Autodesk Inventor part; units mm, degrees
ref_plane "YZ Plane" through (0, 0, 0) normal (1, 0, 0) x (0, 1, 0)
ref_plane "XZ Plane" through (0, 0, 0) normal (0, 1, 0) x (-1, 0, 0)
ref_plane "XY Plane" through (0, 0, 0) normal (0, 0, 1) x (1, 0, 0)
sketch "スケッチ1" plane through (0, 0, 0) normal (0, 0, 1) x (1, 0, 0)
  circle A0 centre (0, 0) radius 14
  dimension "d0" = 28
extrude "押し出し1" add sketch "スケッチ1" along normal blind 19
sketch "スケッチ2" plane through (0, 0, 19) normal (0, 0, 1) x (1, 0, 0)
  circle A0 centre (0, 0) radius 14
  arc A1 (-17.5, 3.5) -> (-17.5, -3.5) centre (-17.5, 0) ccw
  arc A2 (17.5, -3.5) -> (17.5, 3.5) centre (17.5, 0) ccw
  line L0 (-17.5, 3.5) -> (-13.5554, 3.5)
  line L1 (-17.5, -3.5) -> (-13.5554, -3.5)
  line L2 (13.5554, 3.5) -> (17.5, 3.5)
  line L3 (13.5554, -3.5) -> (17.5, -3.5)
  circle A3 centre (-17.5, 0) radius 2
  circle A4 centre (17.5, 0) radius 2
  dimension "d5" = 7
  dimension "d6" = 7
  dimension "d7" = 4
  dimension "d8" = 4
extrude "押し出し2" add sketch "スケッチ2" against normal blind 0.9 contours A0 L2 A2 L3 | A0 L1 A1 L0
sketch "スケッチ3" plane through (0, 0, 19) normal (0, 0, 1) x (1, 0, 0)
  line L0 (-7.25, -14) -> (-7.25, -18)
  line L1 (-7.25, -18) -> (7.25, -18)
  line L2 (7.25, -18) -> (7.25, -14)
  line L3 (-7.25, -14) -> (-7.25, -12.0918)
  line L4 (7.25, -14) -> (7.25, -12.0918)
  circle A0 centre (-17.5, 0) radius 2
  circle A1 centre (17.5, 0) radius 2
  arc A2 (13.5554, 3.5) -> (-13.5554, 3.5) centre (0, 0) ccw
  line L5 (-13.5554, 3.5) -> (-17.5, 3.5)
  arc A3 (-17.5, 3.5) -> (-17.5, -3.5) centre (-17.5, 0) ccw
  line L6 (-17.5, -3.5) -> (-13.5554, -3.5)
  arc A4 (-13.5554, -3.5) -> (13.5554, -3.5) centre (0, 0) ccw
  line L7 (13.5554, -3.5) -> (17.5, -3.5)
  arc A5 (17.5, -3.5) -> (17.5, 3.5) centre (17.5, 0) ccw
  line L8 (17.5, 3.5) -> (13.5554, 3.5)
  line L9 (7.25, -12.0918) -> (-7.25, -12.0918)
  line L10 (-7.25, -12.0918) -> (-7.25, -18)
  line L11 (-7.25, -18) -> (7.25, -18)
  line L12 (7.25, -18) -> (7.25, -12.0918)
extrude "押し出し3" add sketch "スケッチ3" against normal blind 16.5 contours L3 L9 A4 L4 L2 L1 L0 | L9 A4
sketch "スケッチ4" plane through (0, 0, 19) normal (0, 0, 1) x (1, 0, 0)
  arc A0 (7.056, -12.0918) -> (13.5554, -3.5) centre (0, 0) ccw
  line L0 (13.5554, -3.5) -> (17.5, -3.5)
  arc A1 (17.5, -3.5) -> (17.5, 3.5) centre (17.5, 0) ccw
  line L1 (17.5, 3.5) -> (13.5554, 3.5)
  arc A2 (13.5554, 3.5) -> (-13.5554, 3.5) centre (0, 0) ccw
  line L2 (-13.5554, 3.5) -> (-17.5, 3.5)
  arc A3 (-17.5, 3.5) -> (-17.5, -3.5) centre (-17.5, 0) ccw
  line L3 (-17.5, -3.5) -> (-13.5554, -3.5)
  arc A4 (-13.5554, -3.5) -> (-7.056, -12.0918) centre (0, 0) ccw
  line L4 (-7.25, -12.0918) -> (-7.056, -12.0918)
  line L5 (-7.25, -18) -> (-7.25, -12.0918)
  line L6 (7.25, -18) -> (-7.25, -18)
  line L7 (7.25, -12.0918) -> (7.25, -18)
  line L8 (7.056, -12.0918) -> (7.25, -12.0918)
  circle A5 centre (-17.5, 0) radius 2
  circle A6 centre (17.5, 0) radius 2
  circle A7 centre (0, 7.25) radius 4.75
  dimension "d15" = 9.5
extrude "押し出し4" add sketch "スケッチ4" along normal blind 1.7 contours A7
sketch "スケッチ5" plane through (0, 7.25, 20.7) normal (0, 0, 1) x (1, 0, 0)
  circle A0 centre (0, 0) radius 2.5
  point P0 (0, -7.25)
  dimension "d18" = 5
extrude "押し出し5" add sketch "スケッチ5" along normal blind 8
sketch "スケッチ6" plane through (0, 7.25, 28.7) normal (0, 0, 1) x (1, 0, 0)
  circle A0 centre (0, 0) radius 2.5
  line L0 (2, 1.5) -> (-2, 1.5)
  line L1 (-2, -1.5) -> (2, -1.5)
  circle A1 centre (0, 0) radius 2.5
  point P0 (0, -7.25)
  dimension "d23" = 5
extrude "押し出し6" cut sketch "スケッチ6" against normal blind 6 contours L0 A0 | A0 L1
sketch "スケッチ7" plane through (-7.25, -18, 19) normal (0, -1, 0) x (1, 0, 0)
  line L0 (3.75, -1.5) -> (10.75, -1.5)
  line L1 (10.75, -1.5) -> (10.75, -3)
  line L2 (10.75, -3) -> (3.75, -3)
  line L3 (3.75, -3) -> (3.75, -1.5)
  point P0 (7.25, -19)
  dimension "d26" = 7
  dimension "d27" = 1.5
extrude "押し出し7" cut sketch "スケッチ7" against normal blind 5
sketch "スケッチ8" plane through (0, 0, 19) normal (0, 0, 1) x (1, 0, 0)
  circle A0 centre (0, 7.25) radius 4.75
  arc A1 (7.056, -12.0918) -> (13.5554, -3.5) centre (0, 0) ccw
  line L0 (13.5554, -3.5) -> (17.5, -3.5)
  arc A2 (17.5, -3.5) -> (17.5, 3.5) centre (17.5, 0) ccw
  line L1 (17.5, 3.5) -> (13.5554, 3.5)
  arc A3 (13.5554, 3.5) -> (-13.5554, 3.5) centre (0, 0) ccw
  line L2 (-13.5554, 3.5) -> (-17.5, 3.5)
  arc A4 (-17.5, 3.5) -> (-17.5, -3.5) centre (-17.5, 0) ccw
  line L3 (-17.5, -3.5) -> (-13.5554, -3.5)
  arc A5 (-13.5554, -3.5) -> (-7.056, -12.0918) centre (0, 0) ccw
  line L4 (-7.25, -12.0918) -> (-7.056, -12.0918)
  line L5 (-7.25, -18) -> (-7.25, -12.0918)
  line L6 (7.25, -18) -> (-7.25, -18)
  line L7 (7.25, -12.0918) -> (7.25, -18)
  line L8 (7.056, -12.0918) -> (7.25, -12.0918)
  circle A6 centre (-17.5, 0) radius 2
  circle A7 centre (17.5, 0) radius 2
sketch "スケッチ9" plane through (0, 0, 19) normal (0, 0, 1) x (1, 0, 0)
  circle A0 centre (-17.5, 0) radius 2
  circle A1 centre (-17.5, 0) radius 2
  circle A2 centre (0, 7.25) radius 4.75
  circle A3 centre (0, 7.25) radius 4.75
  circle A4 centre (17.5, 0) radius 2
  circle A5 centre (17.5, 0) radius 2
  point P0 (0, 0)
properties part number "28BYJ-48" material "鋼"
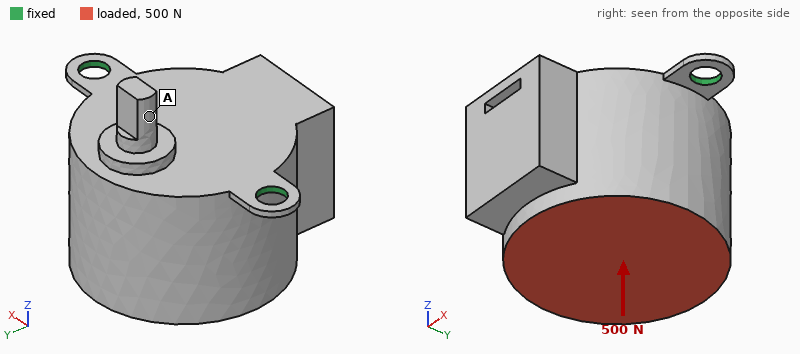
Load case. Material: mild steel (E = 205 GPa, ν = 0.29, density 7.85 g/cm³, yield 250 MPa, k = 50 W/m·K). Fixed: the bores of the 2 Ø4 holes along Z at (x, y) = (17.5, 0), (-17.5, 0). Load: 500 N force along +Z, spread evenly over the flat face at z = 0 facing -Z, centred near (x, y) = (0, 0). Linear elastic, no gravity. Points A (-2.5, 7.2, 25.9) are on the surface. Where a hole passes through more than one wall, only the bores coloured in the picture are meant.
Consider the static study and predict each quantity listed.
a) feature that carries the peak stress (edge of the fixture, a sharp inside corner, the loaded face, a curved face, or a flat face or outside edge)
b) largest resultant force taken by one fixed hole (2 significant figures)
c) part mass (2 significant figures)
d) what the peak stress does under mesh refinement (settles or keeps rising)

edge of the fixture
290 N
100 g
keeps rising
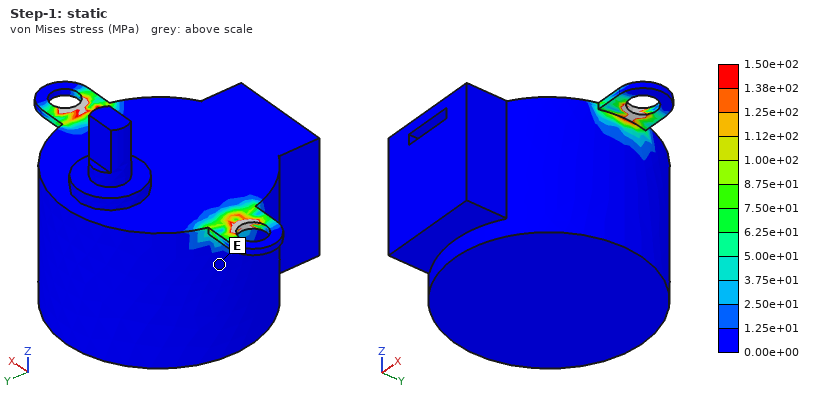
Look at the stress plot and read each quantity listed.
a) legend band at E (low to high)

0.00e+00 to 1.25e+01 MPa
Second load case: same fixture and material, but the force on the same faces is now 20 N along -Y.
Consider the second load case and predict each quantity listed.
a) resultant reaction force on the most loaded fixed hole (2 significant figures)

10 N
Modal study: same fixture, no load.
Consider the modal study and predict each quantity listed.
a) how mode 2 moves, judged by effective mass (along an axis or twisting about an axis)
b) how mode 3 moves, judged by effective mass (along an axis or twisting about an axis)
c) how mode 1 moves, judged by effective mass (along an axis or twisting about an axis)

along Z
along X
along Y
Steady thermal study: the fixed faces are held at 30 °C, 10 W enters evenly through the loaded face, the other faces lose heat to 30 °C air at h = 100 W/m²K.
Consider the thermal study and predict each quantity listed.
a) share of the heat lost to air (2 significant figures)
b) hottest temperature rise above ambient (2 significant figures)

63 %
25 K
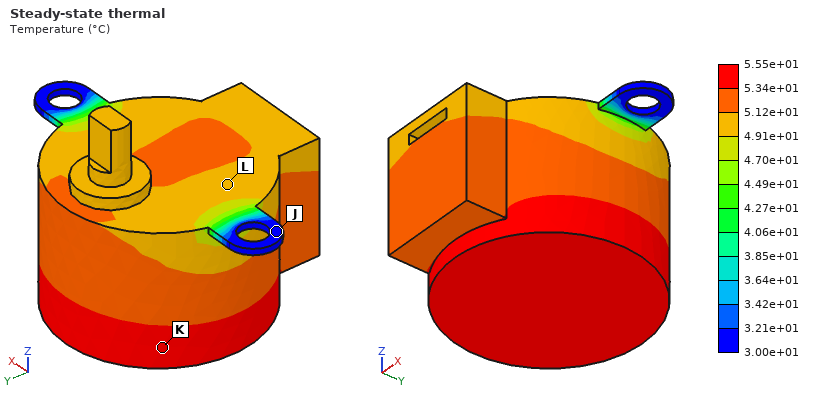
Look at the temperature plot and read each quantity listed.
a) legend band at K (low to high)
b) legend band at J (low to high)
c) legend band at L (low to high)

5.34e+01 to 5.55e+01 °C
3.00e+01 to 3.21e+01 °C
4.91e+01 to 5.12e+01 °C
